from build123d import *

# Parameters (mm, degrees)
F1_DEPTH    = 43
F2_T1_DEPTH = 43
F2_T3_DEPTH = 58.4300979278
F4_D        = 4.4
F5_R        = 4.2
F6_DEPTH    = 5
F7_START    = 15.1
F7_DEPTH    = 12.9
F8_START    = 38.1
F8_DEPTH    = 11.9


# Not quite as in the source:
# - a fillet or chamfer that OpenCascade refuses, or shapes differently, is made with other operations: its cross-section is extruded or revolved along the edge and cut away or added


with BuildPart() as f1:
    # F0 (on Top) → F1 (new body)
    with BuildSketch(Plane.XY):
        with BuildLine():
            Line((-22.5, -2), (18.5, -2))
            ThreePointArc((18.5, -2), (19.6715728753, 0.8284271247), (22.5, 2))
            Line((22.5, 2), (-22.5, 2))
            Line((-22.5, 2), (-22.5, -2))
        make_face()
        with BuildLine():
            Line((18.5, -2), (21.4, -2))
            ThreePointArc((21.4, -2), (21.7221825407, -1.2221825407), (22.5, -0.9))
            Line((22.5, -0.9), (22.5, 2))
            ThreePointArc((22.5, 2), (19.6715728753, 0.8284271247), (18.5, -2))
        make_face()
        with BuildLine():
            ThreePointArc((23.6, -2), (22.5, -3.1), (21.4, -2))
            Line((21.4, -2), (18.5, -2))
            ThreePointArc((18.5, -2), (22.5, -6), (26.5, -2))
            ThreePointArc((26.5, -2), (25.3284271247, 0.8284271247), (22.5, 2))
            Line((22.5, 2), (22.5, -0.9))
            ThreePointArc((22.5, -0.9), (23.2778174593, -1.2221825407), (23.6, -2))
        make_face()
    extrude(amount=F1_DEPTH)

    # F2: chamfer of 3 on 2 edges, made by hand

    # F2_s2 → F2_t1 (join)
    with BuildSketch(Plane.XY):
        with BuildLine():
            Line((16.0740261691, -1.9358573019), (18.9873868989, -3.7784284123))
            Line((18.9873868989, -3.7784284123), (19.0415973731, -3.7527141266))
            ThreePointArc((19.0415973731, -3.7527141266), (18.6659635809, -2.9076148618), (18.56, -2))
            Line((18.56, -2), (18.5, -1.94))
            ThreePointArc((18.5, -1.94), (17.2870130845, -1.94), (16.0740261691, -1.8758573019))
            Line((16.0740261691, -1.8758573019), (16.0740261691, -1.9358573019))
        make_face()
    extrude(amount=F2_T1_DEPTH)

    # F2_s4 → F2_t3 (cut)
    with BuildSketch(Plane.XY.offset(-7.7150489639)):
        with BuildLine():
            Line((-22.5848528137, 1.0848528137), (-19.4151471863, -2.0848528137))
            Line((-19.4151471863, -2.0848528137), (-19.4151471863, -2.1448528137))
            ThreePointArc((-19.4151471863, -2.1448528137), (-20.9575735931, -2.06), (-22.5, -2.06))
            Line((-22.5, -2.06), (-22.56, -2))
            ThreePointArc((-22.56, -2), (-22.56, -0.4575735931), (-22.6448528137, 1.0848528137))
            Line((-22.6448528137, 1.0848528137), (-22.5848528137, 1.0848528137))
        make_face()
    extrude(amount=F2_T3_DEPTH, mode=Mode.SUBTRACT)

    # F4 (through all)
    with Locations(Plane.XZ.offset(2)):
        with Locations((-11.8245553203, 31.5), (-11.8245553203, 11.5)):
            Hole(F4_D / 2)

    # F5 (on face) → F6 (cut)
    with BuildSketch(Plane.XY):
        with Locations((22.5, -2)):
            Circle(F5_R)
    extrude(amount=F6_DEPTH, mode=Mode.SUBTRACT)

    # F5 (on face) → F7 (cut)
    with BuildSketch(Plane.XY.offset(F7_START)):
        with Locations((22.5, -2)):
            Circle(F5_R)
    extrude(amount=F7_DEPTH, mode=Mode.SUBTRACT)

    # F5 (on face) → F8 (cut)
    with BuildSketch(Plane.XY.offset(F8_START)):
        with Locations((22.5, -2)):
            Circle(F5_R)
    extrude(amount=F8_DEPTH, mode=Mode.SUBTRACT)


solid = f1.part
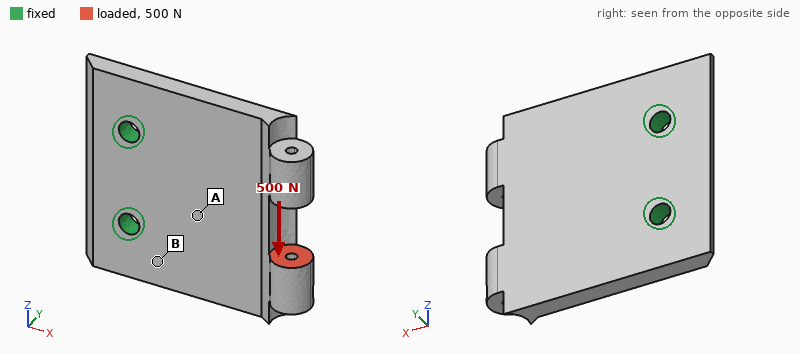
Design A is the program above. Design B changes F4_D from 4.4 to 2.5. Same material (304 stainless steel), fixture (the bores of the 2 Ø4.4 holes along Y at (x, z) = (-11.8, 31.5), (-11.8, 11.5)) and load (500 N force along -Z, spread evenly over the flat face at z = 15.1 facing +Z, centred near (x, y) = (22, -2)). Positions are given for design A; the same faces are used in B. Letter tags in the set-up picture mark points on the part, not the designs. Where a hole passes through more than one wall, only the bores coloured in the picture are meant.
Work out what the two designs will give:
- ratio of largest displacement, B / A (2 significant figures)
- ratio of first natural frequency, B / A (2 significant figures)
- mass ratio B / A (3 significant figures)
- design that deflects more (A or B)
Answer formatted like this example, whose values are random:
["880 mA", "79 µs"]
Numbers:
["1.1", "0.90", "1.01", "B"]
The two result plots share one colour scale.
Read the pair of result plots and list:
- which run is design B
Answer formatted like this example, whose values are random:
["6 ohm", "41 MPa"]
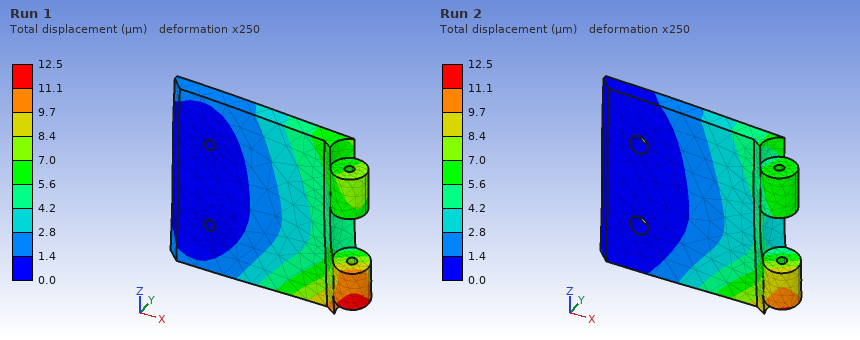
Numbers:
["Run 1"]
